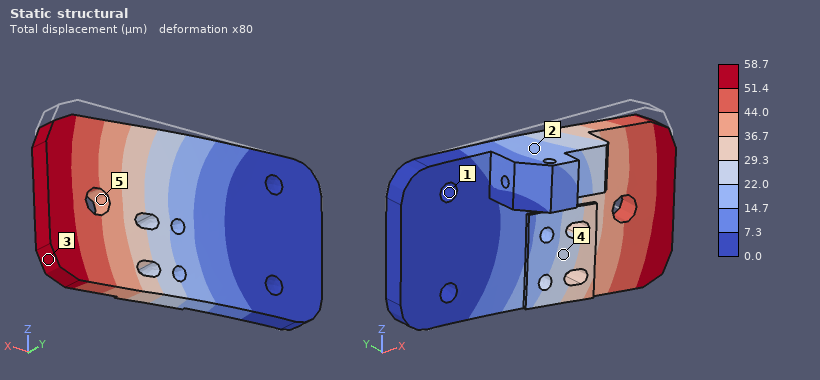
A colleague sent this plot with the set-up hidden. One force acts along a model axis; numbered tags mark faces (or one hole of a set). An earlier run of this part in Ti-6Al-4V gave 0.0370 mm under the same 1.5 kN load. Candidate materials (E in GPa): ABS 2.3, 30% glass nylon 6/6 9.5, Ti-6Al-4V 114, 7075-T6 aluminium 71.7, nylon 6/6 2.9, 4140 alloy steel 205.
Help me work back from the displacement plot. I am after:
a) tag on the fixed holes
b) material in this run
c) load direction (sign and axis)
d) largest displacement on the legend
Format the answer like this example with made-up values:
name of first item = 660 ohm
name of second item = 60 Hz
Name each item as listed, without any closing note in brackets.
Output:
tag on the fixed holes = 1
material in this run = 7075-T6 aluminium
load direction = -Z
largest displacement on the legend = 58.7 µm
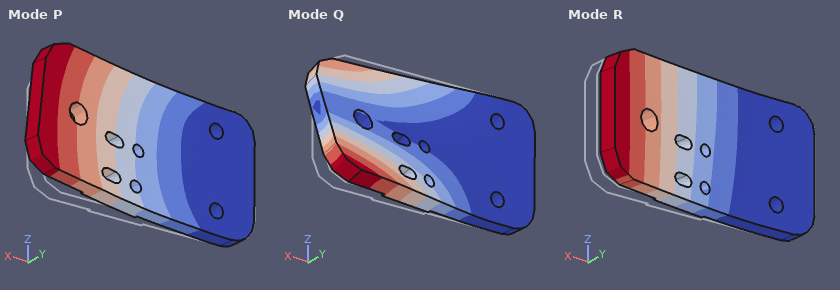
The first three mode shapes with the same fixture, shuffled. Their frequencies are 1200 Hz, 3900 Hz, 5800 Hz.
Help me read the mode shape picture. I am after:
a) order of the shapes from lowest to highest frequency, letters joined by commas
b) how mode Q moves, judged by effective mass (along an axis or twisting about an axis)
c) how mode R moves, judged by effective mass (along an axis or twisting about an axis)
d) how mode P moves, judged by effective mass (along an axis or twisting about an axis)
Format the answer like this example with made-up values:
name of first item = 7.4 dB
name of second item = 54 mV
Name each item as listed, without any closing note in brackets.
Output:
order of the shapes from lowest to highest frequency, letters joined by commas = R, Q, P
how mode Q moves, judged by effective mass = twisting about X
how mode R moves, judged by effective mass = along Y
how mode P moves, judged by effective mass = along Z
